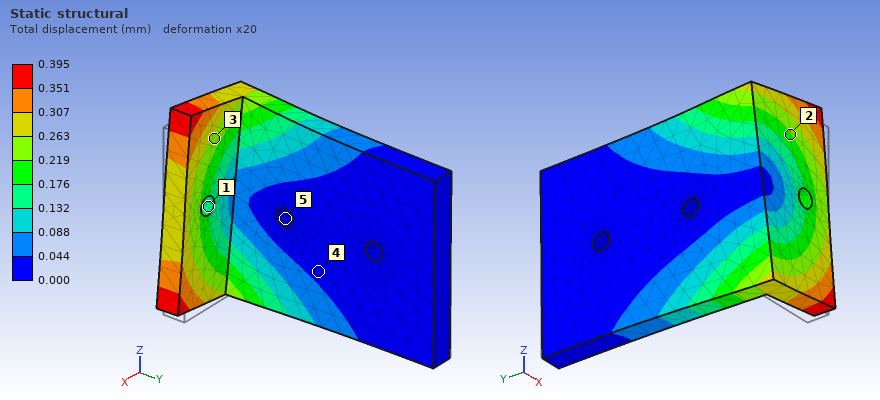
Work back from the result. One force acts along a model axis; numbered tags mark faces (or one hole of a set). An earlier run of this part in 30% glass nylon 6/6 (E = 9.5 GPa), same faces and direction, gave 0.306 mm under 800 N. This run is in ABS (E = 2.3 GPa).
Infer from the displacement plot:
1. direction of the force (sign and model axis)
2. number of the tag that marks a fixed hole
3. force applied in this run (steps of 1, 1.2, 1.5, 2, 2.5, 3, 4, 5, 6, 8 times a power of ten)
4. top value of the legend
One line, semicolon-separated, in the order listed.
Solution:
+Z; 5; 250 N; 0.395 mm
